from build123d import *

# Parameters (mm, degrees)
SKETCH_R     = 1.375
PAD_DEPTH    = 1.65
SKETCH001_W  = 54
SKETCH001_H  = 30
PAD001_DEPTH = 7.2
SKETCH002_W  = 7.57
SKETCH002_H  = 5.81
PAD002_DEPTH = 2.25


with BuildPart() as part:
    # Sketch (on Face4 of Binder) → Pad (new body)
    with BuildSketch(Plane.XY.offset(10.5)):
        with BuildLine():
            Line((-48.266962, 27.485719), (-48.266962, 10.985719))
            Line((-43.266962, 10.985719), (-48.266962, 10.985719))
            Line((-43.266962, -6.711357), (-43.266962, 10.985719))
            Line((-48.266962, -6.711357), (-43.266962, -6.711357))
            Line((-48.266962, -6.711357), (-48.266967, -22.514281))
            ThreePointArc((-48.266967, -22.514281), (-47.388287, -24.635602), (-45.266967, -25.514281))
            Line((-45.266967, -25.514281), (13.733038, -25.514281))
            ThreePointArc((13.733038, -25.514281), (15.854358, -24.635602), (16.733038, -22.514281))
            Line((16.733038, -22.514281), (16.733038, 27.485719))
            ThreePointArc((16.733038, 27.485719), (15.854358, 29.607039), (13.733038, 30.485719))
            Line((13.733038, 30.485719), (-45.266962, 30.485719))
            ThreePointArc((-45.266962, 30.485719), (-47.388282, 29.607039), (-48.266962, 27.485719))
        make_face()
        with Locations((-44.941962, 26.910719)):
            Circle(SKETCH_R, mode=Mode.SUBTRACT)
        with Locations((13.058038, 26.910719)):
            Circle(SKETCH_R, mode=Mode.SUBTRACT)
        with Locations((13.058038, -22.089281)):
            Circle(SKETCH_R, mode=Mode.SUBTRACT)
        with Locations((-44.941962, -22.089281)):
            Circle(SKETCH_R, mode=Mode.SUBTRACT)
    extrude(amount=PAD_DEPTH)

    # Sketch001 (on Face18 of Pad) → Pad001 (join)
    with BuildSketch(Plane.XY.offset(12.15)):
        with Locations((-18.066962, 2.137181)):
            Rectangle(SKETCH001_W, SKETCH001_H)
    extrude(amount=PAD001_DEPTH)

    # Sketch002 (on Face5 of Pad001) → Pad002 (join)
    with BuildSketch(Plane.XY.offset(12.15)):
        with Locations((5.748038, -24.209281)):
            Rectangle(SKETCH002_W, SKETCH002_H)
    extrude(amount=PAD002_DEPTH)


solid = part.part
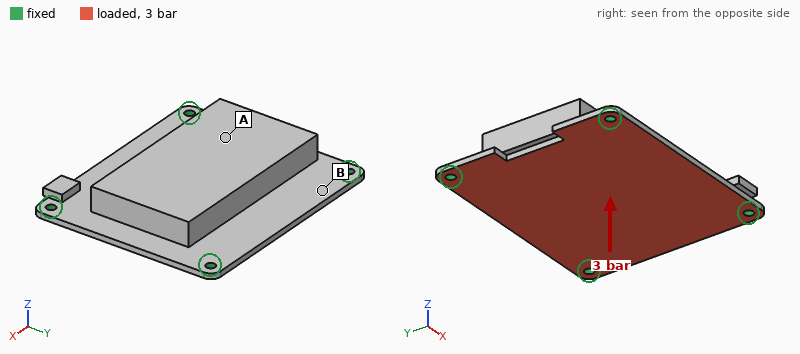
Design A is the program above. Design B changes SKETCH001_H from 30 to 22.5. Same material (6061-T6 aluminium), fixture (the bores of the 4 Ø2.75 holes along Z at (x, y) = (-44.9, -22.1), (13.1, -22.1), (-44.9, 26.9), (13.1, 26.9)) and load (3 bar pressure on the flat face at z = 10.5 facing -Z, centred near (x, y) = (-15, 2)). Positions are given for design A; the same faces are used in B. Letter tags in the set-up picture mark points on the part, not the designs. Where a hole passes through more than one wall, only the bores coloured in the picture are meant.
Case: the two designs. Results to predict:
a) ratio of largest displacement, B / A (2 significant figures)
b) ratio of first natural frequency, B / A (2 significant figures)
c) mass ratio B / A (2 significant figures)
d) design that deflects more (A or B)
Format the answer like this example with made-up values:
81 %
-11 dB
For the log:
1.5
0.82
0.83
B
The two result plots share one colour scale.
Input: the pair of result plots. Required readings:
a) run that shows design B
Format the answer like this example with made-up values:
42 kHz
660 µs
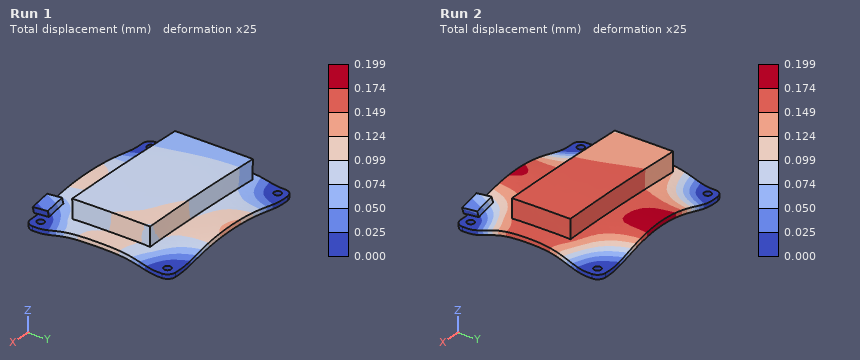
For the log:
Run 2
